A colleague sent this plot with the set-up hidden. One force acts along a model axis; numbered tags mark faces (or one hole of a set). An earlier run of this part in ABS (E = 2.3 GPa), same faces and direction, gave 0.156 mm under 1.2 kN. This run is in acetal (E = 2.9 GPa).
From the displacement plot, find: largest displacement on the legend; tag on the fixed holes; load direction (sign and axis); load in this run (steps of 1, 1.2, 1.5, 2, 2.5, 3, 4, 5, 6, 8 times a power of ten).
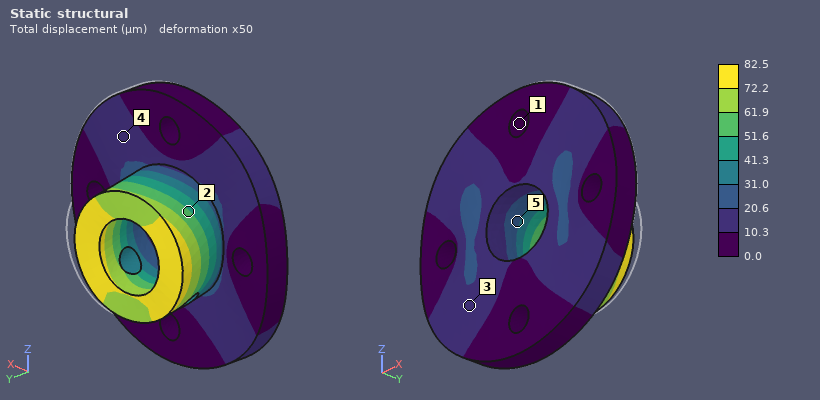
82.5 µm
1
-X
800 N
